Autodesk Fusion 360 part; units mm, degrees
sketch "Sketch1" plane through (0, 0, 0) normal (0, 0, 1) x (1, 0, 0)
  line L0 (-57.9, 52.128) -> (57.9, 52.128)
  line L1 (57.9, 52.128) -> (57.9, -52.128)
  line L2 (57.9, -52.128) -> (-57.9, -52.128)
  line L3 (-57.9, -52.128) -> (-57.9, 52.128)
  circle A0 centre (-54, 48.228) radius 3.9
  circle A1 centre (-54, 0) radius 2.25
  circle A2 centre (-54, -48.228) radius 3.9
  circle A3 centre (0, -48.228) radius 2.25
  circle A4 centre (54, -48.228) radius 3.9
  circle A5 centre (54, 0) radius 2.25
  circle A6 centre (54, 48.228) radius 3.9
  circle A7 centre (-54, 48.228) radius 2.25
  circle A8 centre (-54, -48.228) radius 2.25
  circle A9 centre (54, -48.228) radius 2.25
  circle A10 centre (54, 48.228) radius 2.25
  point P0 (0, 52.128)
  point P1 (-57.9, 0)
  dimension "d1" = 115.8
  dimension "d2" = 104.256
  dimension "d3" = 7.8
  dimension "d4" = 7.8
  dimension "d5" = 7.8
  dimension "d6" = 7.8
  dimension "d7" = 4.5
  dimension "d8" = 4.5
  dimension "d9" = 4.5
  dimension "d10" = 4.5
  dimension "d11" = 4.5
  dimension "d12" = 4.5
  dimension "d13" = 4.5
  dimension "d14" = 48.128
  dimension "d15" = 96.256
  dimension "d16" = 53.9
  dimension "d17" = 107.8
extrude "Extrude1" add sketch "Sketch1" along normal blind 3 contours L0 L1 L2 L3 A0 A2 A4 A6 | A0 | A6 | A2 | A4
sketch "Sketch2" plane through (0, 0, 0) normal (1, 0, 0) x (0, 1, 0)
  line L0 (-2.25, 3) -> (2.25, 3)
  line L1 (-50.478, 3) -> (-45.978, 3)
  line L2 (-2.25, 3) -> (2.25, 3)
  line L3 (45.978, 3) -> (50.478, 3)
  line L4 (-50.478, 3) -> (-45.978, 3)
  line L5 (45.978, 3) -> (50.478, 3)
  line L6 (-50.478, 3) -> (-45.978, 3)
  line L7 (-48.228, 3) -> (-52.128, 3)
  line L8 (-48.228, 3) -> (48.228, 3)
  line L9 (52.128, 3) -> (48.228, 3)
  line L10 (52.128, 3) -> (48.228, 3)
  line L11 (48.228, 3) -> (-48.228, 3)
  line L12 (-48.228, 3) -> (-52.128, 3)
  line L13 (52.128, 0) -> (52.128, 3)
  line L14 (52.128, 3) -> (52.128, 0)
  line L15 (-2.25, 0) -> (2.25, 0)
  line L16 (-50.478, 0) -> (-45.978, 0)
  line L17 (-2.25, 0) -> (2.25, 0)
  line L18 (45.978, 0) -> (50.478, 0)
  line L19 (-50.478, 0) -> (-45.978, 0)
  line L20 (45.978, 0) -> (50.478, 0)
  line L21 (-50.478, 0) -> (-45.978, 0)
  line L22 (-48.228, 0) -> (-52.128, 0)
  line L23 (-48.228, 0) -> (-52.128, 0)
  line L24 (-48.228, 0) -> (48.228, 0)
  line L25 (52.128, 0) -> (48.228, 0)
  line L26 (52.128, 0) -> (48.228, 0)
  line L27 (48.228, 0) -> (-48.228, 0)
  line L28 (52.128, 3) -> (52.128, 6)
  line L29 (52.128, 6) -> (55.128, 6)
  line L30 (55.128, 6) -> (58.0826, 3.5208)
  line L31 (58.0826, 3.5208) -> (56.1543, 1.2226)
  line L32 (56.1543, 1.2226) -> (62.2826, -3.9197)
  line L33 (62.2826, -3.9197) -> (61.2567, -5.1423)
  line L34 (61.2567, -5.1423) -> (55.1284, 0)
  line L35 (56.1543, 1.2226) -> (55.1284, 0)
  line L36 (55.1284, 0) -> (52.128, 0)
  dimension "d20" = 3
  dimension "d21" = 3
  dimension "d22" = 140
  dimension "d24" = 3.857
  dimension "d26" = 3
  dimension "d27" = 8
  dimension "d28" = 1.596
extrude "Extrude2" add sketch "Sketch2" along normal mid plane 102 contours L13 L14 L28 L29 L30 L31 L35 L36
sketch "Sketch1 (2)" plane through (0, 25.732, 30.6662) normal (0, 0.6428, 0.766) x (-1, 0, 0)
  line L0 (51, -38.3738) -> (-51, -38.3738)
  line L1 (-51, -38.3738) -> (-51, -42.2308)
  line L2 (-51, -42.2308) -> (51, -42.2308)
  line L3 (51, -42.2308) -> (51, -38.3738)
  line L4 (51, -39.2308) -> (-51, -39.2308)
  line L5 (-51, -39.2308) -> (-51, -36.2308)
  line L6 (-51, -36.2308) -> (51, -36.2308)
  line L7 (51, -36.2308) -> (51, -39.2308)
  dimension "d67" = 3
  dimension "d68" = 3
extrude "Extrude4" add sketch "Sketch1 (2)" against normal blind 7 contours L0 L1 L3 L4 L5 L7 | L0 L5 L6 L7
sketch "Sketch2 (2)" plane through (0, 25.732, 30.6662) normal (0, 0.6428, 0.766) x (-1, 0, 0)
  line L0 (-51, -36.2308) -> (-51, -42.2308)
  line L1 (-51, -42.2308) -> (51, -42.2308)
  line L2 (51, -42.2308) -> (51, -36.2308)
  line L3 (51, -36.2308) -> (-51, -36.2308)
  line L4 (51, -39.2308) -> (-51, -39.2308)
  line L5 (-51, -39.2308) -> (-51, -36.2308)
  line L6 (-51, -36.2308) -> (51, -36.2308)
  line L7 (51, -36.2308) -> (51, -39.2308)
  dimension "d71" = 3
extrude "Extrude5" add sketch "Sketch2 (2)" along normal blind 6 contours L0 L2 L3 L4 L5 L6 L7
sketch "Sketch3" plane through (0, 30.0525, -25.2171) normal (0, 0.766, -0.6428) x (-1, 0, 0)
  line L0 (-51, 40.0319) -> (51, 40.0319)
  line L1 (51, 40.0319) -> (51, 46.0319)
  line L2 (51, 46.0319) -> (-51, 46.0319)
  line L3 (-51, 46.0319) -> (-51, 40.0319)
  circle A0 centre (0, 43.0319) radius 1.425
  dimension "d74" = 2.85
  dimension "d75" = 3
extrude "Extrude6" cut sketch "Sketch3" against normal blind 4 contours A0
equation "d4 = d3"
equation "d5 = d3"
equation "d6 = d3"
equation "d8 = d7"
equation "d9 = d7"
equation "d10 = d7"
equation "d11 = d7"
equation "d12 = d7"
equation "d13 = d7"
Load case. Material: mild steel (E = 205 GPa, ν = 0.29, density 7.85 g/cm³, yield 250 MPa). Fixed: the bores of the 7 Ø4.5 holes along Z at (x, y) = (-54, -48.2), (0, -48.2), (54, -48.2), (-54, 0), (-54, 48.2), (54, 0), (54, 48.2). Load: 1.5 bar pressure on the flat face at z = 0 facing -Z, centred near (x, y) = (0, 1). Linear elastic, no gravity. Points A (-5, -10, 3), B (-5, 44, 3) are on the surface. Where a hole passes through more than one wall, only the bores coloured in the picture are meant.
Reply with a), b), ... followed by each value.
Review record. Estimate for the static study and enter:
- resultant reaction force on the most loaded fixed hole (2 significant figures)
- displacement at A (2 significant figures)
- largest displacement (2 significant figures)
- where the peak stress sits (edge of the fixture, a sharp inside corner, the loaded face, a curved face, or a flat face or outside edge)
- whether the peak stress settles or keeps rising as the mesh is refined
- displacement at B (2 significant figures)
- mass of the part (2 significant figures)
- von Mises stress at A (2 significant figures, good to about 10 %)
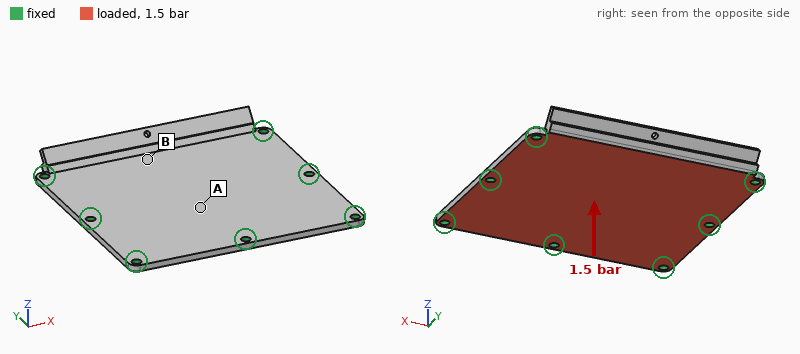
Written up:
a) 500 N
b) 65 µm
c) 77 µm
d) edge of the fixture
e) keeps rising
f) 43 µm
g) 320 g
h) 25 MPa
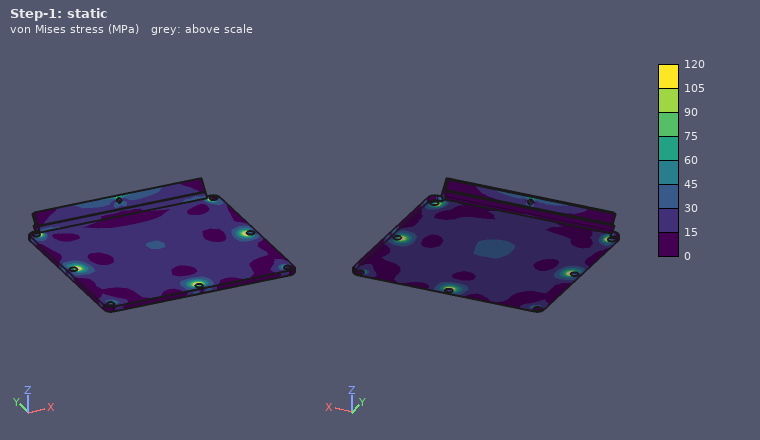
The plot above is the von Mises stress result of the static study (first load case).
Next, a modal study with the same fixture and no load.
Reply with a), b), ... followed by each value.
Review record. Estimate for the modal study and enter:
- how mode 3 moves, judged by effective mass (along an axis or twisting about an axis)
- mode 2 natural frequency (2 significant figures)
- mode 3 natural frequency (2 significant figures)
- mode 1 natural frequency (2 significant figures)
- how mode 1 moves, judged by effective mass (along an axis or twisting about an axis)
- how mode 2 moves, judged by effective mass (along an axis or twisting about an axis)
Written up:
a) twisting about Y
b) 2700 Hz
c) 3700 Hz
d) 1800 Hz
e) along Z
f) twisting about X
